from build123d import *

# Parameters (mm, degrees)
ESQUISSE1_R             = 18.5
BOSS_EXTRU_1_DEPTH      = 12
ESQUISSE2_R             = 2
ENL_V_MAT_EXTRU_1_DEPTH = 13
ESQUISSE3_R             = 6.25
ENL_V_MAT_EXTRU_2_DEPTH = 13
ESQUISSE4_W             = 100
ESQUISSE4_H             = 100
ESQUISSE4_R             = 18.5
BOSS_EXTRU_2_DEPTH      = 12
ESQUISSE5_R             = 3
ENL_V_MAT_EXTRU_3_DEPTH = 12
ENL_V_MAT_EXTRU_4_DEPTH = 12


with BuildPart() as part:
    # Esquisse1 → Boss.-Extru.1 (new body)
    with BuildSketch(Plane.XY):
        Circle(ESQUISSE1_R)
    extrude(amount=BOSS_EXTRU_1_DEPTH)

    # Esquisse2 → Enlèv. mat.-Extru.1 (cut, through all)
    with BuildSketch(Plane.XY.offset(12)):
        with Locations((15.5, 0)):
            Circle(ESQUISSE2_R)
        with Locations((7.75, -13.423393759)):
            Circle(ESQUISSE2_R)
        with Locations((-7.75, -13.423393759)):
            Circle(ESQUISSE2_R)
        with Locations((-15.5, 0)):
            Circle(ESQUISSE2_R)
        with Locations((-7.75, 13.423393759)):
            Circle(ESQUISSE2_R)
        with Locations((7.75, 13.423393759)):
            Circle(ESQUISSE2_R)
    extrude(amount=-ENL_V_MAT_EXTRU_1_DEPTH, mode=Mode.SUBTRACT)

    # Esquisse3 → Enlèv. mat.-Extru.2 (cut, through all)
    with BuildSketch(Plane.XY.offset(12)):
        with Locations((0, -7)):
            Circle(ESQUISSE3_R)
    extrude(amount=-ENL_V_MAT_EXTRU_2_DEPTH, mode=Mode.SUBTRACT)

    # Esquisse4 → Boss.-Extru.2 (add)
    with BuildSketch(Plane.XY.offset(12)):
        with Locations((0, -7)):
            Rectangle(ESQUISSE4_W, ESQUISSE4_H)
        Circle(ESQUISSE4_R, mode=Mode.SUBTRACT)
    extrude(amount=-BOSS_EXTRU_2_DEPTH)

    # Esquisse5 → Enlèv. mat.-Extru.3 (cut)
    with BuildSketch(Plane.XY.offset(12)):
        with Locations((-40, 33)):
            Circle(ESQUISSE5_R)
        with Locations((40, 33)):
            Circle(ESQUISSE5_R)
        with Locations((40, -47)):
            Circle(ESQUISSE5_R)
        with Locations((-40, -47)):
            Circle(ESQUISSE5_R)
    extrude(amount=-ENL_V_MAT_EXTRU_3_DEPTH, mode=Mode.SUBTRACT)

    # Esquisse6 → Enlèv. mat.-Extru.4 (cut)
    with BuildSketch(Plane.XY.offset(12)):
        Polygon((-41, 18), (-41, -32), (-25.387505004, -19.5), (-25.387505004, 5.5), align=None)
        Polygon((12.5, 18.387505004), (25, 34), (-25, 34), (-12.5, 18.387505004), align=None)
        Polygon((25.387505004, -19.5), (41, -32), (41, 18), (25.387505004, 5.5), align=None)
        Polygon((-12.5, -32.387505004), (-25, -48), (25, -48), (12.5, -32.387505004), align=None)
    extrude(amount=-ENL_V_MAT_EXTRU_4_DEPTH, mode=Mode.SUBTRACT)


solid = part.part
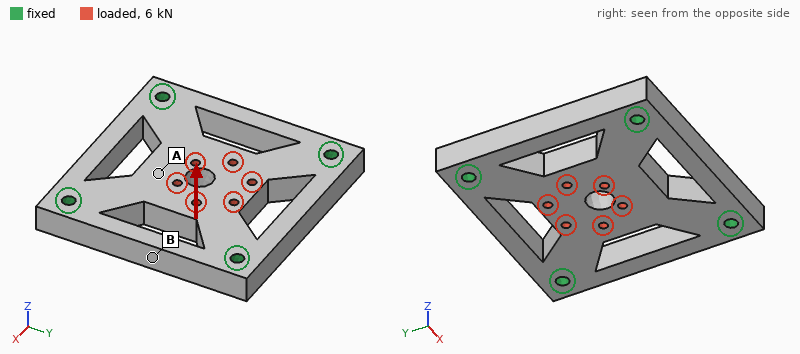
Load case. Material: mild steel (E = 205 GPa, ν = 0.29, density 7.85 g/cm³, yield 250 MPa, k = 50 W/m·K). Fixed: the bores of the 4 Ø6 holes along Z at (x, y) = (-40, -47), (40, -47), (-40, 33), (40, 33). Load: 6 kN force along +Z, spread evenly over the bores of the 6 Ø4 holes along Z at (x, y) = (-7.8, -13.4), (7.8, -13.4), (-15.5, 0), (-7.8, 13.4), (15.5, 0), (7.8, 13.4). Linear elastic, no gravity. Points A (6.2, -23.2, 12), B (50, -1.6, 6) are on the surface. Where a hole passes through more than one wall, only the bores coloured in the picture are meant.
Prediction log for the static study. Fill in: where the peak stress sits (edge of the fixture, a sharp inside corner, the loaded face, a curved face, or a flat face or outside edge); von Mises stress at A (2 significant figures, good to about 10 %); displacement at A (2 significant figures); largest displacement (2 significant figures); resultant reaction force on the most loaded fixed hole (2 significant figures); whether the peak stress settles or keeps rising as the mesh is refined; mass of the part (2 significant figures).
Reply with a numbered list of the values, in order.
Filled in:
1. edge of the fixture
2. 29 MPa
3. 20 µm
4. 27 µm
5. 1.8 kN
6. keeps rising
7. 690 g
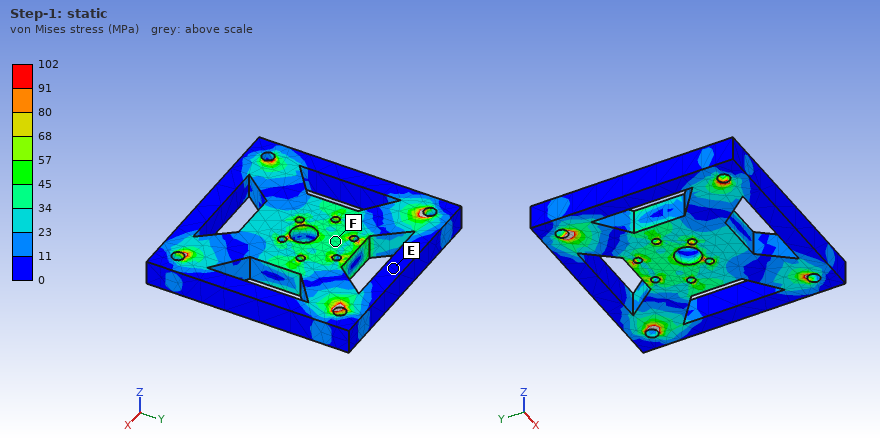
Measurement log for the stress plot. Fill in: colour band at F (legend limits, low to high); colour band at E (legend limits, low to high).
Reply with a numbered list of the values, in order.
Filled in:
1. 34 to 45 MPa
2. 0 to 11 MPa
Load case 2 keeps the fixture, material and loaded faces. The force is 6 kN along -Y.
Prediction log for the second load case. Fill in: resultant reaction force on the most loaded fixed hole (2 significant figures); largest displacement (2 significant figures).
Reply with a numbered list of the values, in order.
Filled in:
1. 1.8 kN
2. 2.9 µm
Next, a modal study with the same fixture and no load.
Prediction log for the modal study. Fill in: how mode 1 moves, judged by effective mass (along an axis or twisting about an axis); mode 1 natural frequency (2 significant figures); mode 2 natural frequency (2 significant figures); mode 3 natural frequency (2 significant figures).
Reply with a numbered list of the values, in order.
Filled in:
1. along Z
2. 5600 Hz
3. 9900 Hz
4. 9900 Hz
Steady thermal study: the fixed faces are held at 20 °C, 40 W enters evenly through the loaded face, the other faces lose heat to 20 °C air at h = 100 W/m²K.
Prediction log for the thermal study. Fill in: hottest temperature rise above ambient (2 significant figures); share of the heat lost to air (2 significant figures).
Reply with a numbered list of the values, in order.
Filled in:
1. 25 K
2. 45 %
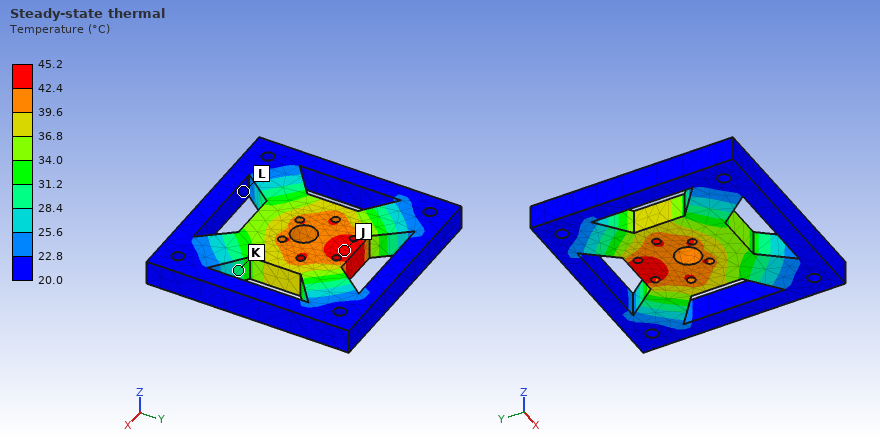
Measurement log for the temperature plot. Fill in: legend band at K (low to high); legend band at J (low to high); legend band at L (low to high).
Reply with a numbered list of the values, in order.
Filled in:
1. 28.4 to 31.2 °C
2. 42.4 to 45.2 °C
3. 20.0 to 22.8 °C
